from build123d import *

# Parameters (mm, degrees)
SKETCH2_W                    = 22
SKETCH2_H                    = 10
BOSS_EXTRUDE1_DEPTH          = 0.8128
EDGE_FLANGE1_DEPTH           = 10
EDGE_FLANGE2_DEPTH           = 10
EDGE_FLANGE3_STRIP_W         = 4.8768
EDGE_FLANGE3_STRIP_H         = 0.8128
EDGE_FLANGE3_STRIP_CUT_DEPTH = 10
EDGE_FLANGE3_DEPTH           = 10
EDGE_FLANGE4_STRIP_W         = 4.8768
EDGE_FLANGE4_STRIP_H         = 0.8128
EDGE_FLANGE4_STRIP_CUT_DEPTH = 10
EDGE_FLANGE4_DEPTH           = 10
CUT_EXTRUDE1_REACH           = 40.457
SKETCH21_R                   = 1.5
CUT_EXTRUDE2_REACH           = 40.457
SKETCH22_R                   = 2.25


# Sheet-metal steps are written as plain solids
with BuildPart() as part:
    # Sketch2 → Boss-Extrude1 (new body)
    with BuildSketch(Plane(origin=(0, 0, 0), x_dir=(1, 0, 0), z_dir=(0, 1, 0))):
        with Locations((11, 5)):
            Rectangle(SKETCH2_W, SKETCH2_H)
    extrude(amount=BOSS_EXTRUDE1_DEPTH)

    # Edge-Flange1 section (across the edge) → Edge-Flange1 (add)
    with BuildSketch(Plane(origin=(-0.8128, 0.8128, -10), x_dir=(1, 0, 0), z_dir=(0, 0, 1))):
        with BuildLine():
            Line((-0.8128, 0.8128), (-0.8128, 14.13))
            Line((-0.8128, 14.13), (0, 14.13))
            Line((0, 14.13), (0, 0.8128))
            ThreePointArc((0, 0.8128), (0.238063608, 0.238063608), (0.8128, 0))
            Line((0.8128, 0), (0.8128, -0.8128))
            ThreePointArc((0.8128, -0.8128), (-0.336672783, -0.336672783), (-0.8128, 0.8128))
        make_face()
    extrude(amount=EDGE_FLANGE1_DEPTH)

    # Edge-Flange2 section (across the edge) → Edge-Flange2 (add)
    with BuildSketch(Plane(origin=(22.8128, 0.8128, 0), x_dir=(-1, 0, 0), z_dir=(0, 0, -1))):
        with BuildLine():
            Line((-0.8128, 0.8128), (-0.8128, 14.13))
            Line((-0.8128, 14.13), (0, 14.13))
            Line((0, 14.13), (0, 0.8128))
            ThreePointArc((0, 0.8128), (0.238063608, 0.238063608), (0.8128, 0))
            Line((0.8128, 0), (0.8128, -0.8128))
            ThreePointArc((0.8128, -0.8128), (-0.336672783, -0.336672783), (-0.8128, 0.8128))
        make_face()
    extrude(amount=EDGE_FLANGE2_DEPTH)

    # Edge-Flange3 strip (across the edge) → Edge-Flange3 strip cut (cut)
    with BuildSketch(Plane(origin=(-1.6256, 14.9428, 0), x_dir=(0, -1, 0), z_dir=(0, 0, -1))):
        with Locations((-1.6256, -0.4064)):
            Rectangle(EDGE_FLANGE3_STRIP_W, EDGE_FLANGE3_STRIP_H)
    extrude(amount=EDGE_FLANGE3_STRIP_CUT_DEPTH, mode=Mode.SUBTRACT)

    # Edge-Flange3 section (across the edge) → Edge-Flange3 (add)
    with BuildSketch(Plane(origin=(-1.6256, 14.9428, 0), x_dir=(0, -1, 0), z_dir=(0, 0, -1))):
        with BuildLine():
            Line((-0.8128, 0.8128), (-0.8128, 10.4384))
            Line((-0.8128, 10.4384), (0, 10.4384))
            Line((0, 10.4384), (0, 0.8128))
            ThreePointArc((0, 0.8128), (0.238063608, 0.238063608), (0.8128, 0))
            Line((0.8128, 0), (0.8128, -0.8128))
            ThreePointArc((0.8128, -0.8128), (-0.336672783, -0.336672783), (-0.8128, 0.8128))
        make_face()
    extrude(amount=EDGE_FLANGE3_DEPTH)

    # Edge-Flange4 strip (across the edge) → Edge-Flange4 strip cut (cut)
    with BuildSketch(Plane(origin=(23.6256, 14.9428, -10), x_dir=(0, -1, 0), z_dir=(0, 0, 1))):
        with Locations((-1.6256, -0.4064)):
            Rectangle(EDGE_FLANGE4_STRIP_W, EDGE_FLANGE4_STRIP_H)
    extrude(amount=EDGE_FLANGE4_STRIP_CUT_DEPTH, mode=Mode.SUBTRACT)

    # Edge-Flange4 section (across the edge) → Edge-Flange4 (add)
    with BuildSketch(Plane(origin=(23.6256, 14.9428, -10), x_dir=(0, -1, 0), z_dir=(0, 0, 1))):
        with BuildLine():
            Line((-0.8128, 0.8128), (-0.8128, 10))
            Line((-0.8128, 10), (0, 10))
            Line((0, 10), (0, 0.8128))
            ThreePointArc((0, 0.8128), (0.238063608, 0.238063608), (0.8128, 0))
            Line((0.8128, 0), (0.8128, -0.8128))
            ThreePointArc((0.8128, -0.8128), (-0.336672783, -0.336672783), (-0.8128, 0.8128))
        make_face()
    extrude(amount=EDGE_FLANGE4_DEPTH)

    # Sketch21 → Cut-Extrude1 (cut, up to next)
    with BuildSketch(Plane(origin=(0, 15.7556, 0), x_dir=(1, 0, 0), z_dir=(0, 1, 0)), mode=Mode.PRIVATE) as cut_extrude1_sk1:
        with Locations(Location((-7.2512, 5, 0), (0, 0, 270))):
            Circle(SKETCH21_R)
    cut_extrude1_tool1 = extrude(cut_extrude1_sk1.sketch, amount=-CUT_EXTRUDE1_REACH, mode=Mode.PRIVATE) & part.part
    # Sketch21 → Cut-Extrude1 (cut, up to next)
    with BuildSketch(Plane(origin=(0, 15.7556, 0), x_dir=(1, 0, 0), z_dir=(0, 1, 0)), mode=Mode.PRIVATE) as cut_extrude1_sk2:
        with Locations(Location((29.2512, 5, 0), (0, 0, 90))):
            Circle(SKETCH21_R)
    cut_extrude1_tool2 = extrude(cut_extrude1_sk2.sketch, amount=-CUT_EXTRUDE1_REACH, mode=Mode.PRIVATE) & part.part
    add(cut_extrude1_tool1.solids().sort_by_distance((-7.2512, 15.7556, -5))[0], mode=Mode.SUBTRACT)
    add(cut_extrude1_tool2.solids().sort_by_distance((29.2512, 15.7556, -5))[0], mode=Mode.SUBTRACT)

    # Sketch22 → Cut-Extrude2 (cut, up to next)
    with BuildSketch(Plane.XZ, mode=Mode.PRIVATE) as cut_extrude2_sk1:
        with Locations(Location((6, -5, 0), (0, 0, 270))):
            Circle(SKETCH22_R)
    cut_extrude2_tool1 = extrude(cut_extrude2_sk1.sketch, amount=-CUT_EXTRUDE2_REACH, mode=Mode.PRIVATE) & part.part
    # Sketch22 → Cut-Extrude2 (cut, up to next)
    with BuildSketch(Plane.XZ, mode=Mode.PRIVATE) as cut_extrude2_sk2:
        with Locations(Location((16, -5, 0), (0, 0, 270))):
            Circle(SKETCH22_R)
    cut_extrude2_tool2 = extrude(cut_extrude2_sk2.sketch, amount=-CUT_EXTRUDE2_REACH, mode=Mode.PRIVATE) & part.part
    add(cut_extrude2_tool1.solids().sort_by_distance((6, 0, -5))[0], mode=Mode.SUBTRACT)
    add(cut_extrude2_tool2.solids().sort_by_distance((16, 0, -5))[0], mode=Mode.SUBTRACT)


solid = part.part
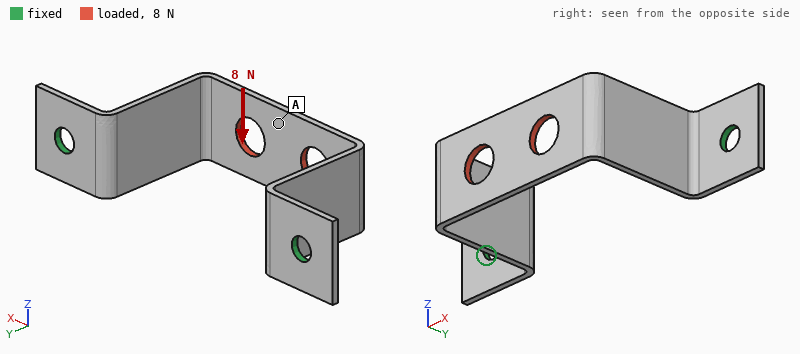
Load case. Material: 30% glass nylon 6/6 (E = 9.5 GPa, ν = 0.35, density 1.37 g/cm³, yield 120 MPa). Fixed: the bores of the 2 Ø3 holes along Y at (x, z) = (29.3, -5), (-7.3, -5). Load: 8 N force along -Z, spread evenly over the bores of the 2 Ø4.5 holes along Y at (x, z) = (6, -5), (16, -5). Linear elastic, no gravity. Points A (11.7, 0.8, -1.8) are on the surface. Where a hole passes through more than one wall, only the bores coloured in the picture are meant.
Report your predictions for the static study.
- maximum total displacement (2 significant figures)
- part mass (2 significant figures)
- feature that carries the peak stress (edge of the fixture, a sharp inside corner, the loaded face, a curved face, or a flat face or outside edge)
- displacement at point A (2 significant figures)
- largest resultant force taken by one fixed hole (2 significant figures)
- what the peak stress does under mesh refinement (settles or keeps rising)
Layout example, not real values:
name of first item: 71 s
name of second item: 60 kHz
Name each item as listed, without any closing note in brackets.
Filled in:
maximum total displacement: 0.52 mm
part mass: 0.77 g
feature that carries the peak stress: edge of the fixture
displacement at point A: 0.48 mm
largest resultant force taken by one fixed hole: 4.0 N
what the peak stress does under mesh refinement: keeps rising
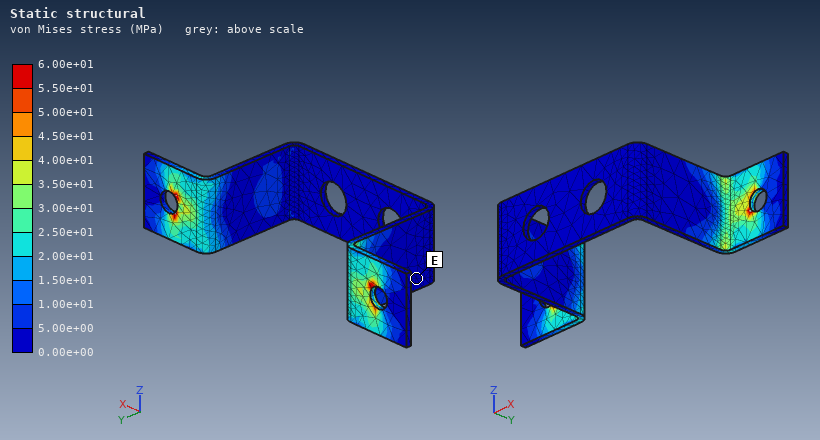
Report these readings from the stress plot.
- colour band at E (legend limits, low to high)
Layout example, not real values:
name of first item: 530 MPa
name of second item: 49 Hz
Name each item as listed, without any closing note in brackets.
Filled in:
colour band at E: 0.00e+00 to 5.00e+00 MPa
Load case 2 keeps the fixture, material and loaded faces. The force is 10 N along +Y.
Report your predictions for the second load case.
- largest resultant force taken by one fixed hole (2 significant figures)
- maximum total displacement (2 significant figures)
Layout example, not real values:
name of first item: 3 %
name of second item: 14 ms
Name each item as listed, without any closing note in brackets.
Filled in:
largest resultant force taken by one fixed hole: 5.5 N
maximum total displacement: 0.23 mm
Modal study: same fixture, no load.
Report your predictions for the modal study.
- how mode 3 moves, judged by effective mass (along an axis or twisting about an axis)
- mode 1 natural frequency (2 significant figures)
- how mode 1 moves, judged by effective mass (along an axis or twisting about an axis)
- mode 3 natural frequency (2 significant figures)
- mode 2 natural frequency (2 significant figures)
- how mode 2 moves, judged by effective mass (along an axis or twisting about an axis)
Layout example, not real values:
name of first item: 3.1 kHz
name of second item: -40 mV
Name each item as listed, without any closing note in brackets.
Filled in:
how mode 3 moves, judged by effective mass: twisting about Y
mode 1 natural frequency: 990 Hz
how mode 1 moves, judged by effective mass: along X
mode 3 natural frequency: 1700 Hz
mode 2 natural frequency: 1100 Hz
how mode 2 moves, judged by effective mass: along Z
